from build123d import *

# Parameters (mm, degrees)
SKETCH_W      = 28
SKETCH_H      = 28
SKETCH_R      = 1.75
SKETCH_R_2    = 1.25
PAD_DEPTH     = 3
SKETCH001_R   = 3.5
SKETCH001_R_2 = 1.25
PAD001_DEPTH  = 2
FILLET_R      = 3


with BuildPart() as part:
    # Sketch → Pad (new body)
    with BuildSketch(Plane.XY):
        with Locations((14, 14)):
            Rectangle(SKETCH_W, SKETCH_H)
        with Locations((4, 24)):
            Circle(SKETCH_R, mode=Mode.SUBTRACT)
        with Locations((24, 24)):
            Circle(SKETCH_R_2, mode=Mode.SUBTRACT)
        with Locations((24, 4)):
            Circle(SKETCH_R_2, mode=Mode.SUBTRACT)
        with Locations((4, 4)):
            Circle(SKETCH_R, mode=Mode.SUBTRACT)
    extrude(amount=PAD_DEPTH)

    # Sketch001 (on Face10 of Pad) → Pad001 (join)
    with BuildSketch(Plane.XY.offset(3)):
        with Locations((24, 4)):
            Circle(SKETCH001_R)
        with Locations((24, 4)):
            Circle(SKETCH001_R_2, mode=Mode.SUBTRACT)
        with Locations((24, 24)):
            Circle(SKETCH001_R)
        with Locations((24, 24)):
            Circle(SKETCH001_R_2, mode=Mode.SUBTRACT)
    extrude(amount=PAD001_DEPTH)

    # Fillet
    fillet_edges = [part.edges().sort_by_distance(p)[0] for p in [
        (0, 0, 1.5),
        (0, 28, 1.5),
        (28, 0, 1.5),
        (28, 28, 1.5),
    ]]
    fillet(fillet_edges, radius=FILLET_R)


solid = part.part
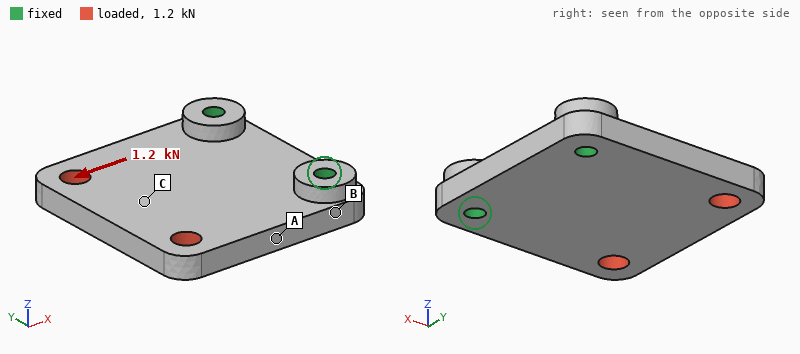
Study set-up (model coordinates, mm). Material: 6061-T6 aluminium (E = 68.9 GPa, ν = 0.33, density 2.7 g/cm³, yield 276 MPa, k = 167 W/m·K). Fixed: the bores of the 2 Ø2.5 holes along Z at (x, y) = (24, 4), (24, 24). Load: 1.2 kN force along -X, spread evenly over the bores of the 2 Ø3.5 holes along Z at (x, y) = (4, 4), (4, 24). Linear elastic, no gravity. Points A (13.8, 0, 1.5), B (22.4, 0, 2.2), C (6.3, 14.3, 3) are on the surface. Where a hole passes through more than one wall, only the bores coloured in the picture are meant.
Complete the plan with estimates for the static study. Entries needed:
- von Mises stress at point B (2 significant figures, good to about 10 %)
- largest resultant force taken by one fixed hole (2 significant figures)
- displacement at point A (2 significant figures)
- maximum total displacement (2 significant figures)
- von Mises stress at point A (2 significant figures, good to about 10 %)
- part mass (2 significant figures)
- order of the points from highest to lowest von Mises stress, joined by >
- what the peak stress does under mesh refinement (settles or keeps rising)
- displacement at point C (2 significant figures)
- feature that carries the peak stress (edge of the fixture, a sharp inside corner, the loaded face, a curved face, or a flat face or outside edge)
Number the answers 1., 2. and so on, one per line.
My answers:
1. 11 MPa
2. 610 N
3. 3.6 µm
4. 9.1 µm
5. 22 MPa
6. 6.4 g
7. A > B > C
8. keeps rising
9. 4.4 µm
10. edge of the fixture
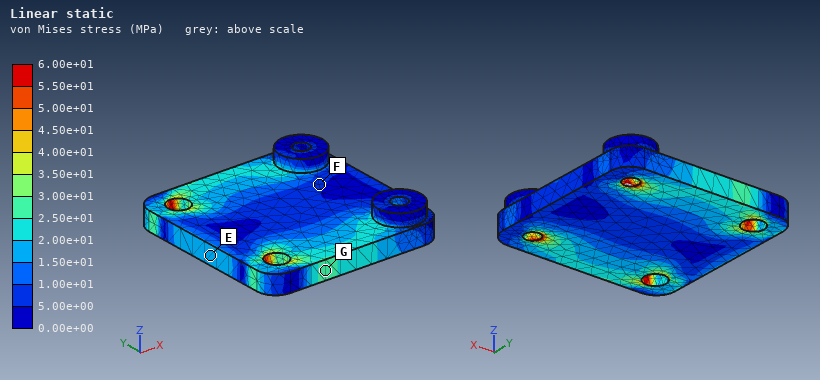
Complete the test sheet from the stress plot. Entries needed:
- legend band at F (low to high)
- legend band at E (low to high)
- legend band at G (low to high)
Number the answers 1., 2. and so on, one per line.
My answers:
1. 5.00e+00 to 1.00e+01 MPa
2. 1.50e+01 to 2.00e+01 MPa
3. 2.50e+01 to 3.00e+01 MPa
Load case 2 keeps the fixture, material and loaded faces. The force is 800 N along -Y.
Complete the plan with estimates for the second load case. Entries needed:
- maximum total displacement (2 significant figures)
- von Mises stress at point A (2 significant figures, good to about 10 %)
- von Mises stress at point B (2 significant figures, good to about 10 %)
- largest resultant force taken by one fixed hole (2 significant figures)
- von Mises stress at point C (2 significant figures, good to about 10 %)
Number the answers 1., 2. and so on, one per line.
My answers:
1. 19 µm
2. 20 MPa
3. 31 MPa
4. 840 N
5. 19 MPa
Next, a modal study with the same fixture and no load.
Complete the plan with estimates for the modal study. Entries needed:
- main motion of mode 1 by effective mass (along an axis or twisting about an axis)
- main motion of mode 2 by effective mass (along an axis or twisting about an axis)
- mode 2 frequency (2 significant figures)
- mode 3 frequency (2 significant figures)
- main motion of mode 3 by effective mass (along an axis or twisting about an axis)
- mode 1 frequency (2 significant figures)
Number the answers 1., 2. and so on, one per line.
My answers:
1. along Z
2. twisting about X
3. 10 kHz
4. 23 kHz
5. along Y
6. 4600 Hz
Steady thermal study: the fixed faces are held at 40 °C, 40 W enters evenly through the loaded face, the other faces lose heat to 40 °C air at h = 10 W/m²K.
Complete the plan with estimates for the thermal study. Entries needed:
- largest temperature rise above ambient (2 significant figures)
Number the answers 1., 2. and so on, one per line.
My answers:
1. 72 K
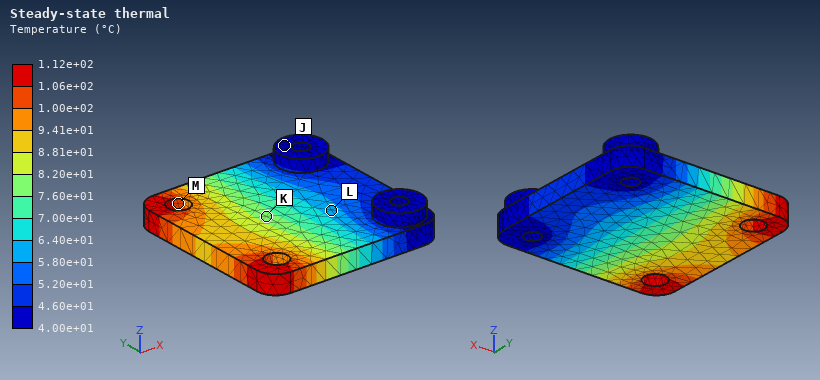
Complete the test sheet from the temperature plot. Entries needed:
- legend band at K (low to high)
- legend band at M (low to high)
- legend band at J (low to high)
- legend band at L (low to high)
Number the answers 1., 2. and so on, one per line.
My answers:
1. 7.60e+01 to 8.20e+01 °C
2. 1.00e+02 to 1.06e+02 °C
3. 4.00e+01 to 4.60e+01 °C
4. 5.80e+01 to 6.40e+01 °C
